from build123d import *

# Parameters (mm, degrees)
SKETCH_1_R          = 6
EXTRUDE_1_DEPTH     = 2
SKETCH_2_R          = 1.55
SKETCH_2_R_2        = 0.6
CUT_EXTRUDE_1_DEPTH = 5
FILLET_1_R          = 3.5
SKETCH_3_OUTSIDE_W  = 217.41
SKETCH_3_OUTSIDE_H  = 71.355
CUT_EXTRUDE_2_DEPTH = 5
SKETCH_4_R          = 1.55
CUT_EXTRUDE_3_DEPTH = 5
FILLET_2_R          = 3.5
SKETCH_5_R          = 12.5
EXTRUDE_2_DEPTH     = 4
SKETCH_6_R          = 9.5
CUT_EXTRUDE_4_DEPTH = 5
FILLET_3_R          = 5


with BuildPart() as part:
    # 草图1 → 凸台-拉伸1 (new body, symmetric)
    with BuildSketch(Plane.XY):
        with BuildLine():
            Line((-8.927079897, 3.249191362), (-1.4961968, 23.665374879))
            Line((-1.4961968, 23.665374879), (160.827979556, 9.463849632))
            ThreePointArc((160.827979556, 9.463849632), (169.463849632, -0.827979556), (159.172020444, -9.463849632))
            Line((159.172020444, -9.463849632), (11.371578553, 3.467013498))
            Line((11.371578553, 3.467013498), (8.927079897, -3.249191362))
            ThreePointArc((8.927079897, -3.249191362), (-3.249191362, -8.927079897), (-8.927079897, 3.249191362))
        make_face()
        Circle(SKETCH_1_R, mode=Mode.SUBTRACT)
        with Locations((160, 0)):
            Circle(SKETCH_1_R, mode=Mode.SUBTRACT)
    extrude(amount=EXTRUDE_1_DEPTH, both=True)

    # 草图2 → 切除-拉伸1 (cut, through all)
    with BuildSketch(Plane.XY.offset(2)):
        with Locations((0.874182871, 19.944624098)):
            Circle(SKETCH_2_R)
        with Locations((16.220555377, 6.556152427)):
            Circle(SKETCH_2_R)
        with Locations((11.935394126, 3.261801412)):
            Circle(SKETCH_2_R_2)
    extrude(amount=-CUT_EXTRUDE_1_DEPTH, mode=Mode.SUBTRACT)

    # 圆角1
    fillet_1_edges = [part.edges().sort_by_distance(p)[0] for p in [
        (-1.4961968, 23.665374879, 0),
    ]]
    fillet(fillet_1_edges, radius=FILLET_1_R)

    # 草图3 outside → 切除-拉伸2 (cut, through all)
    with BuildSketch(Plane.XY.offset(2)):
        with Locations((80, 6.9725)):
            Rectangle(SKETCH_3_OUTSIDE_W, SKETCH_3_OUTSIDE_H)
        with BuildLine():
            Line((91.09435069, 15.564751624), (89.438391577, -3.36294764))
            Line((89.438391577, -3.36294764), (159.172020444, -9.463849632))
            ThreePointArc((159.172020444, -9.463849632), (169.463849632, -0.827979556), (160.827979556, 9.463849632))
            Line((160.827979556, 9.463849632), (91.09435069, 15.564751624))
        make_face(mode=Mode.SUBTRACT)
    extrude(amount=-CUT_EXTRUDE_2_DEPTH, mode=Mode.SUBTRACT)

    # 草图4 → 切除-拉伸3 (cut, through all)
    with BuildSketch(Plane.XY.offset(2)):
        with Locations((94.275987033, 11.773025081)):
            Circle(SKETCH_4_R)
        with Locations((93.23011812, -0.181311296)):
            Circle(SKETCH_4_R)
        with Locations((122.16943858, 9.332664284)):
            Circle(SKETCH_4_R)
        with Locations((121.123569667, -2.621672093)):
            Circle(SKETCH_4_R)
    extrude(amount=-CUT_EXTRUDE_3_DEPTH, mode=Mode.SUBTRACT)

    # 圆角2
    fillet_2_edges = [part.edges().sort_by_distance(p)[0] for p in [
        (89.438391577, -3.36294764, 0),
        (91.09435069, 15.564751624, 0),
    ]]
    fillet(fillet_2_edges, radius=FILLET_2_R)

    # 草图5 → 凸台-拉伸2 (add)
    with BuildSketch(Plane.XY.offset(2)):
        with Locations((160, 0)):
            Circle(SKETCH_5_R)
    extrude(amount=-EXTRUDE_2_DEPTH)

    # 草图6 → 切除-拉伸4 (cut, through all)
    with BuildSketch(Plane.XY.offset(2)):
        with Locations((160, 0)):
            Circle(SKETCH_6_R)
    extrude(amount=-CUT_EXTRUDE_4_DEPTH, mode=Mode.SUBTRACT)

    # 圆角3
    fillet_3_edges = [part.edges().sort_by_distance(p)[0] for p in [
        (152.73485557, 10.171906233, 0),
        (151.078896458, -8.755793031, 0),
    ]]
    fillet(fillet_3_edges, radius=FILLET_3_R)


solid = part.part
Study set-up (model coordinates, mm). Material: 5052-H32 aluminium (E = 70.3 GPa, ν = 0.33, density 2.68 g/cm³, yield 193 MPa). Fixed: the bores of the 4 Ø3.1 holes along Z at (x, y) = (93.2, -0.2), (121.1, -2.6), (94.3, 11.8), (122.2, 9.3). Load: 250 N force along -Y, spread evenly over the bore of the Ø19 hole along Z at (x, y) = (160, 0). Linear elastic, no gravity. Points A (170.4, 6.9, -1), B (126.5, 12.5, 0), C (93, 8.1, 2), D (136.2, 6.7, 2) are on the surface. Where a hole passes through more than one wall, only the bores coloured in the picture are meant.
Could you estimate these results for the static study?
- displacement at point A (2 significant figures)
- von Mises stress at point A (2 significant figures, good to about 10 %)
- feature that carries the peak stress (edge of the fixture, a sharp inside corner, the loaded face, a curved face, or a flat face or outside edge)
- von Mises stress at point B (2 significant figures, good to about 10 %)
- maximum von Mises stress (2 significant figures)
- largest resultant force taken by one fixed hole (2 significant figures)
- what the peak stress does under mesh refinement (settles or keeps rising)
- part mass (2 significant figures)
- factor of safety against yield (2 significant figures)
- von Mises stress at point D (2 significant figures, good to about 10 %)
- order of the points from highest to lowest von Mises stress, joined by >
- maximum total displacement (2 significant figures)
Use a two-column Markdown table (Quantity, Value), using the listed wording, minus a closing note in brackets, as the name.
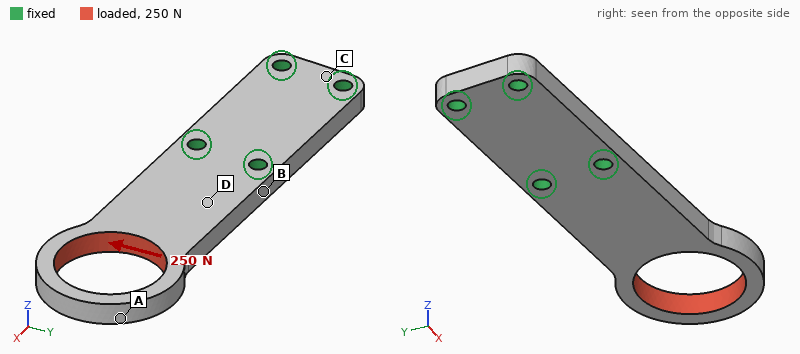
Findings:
| Quantity | Value |
|---|---|
| displacement at point A | 0.11 mm |
| von Mises stress at point A | 37 MPa |
| feature that carries the peak stress | a curved face |
| von Mises stress at point B | 30 MPa |
| maximum von Mises stress | 97 MPa |
| largest resultant force taken by one fixed hole | 700 N |
| what the peak stress does under mesh refinement | settles |
| part mass | 14 g |
| factor of safety against yield | 2.0 |
| von Mises stress at point D | 14 MPa |
| order of the points from highest to lowest von Mises stress, joined by > | A > B > D > C |
| maximum total displacement | 0.11 mm |
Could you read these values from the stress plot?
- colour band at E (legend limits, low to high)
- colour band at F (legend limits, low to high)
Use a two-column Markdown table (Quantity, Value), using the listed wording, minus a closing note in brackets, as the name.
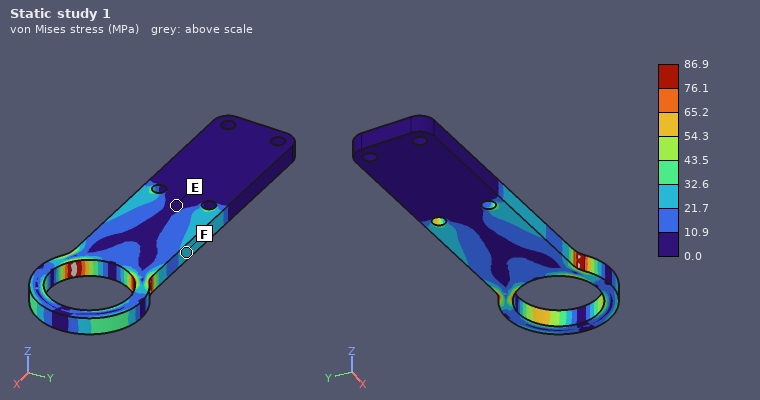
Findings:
| Quantity | Value |
|---|---|
| colour band at E | 0.0 to 10.9 MPa |
| colour band at F | 21.7 to 32.6 MPa |
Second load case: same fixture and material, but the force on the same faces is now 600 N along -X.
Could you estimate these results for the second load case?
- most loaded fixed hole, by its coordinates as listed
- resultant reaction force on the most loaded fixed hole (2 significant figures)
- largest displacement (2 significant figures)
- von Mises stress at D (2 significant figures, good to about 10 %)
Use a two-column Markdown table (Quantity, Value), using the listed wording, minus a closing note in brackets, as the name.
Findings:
| Quantity | Value |
|---|---|
| most loaded fixed hole, by its coordinates as listed | (121.1, -2.6) |
| resultant reaction force on the most loaded fixed hole | 440 N |
| largest displacement | 38 µm |
| von Mises stress at D | 5.8 MPa |
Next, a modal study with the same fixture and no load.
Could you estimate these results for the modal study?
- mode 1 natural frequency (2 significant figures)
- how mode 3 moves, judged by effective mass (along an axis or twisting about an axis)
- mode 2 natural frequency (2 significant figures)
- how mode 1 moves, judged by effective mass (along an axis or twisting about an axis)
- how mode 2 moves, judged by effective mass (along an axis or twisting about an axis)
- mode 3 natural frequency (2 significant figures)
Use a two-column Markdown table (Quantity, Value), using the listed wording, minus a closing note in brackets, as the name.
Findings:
| Quantity | Value |
|---|---|
| mode 1 natural frequency | 1800 Hz |
| how mode 3 moves, judged by effective mass | twisting about X |
| mode 2 natural frequency | 5500 Hz |
| how mode 1 moves, judged by effective mass | along Z |
| how mode 2 moves, judged by effective mass | along Y |
| mode 3 natural frequency | 5900 Hz |
